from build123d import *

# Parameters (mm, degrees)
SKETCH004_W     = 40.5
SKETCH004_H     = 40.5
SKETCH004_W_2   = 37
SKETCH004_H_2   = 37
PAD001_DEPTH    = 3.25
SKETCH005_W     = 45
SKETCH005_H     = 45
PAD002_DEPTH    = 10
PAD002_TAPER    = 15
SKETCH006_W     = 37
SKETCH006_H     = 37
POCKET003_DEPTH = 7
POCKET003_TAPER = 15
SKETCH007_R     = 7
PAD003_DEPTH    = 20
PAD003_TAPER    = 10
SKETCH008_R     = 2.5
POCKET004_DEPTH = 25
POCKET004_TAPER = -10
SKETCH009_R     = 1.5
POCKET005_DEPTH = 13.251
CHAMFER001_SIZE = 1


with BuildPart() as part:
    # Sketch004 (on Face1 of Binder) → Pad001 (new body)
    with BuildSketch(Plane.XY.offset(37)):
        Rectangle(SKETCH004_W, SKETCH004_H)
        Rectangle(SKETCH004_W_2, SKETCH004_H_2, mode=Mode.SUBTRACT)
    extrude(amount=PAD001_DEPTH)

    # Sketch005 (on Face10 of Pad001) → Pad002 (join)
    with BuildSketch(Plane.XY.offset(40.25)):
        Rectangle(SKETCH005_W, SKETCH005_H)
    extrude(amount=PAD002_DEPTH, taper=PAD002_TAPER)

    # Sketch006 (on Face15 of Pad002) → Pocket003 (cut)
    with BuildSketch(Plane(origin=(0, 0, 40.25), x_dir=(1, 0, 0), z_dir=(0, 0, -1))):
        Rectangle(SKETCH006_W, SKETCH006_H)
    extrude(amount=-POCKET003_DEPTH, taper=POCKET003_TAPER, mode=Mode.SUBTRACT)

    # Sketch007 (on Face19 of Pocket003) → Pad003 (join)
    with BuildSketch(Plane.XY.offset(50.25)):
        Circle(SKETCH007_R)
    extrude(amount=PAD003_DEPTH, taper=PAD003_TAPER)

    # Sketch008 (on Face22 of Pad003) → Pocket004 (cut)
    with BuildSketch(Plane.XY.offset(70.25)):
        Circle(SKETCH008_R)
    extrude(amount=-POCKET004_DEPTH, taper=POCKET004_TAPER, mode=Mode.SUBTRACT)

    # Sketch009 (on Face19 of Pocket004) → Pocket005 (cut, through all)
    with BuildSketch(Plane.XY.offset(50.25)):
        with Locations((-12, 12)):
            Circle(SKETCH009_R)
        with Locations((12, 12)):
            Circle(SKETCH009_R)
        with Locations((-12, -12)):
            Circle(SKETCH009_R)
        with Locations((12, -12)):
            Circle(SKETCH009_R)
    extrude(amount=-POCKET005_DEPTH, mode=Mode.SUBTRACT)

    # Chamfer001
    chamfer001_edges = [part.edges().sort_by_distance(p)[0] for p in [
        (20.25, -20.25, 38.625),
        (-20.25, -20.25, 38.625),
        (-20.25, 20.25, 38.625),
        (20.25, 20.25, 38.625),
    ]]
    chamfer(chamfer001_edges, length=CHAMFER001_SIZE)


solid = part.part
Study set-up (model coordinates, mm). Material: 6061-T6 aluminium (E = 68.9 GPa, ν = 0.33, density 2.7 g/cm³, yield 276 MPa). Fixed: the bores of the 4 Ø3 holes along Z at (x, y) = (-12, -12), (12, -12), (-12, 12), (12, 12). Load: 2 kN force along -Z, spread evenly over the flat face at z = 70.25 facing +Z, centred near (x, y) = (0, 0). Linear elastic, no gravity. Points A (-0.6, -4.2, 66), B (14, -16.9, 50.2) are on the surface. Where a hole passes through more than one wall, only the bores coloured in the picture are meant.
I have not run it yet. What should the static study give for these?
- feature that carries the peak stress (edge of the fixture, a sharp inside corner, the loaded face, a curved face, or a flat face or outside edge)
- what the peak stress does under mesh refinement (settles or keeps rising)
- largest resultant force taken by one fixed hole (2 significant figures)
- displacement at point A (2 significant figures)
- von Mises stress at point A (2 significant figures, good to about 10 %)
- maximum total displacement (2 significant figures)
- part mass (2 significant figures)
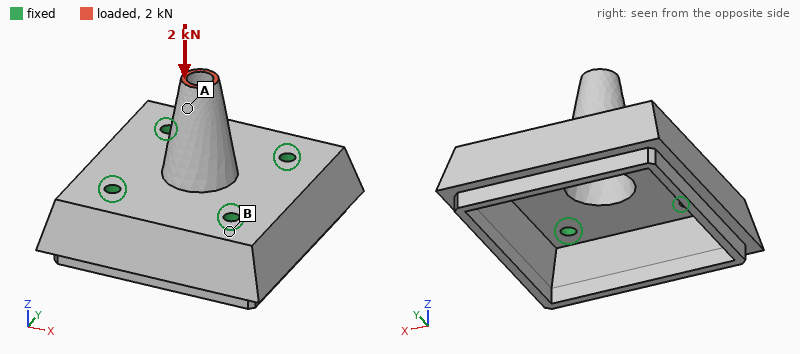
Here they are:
edge of the fixture
keeps rising
520 N
55 µm
90 MPa
64 µm
28 g
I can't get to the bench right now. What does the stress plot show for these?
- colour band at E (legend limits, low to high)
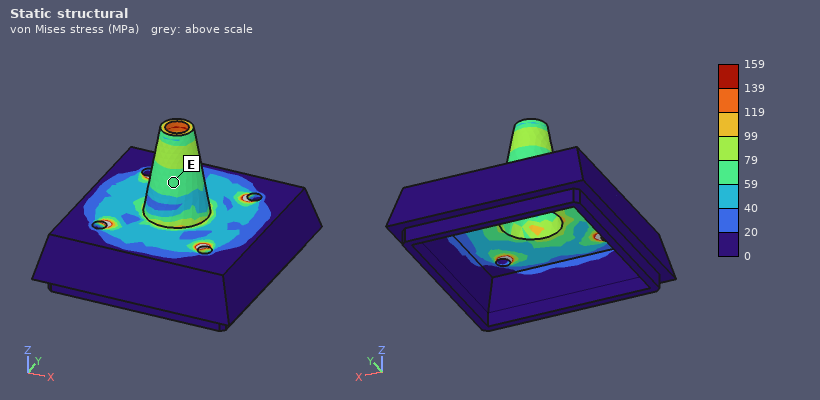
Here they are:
59 to 79 MPa
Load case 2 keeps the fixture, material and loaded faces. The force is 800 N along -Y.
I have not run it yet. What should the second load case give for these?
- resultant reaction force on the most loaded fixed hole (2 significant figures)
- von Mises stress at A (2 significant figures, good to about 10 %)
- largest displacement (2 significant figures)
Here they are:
480 N
96 MPa
0.22 mm
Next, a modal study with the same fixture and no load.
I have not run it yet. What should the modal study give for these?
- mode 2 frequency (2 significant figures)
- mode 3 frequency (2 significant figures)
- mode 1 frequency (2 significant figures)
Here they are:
13 kHz
14 kHz
13 kHz
